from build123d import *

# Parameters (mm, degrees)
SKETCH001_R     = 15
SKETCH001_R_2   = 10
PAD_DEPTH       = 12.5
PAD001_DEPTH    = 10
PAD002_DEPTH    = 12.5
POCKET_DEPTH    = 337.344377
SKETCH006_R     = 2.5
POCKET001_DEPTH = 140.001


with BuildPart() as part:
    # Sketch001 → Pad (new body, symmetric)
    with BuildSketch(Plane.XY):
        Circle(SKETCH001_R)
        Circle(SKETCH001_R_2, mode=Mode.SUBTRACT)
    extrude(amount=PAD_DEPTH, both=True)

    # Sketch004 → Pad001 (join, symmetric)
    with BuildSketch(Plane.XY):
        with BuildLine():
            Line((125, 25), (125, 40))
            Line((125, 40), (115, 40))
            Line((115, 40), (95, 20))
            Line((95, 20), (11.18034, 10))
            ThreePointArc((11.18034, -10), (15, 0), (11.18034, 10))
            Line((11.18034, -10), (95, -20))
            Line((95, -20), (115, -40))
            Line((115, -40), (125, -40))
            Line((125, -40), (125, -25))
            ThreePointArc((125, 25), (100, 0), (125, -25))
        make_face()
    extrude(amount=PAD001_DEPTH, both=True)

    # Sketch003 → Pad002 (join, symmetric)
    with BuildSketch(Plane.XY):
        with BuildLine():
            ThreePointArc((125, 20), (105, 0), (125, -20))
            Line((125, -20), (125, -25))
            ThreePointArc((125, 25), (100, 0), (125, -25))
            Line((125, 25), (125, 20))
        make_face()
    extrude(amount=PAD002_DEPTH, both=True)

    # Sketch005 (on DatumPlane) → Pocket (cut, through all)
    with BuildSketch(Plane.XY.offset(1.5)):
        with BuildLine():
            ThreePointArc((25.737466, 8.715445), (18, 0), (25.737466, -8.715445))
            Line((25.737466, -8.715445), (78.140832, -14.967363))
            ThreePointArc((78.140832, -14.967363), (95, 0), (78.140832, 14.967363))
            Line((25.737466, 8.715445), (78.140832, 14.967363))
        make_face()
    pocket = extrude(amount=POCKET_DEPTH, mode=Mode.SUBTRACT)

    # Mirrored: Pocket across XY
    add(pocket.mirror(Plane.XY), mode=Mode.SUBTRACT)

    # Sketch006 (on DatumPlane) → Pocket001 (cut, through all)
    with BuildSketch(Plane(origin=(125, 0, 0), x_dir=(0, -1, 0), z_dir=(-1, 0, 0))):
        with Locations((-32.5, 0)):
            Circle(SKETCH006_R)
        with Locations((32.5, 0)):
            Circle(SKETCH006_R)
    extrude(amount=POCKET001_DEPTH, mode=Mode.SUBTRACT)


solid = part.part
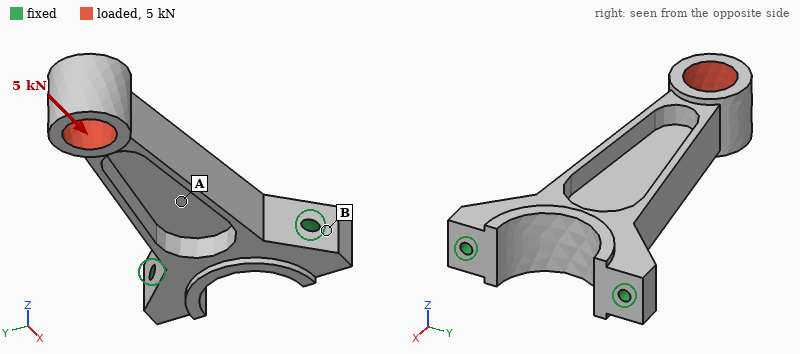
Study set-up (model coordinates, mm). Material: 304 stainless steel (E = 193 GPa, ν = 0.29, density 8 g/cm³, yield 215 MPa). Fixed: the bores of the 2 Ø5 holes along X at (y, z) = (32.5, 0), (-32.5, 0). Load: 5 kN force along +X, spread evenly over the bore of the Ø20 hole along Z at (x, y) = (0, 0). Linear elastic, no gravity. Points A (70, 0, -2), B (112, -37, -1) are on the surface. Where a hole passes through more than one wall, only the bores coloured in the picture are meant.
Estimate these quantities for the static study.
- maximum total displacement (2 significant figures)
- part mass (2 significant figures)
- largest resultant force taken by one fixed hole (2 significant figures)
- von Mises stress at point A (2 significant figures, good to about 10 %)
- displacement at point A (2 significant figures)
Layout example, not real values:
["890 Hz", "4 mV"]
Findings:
["19 µm", "460 g", "3.0 kN", "24 MPa", "5.1 µm"]
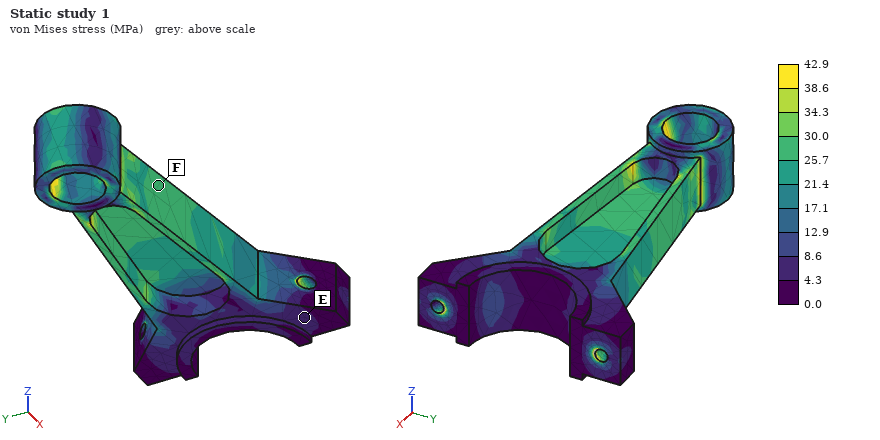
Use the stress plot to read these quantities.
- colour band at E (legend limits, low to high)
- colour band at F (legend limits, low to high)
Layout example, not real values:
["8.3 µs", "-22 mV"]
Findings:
["4.3 to 8.6 MPa", "25.7 to 30.0 MPa"]
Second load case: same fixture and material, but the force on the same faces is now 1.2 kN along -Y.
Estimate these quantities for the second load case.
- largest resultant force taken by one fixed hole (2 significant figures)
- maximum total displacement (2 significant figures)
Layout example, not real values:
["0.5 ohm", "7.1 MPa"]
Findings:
["2.7 kN", "96 µm"]
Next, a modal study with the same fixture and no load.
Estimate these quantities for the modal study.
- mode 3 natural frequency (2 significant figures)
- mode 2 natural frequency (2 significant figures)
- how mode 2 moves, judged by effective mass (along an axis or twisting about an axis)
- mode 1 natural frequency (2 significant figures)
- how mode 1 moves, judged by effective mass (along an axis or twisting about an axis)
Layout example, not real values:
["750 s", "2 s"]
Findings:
["2300 Hz", "1900 Hz", "along Y", "750 Hz", "along Z"]
